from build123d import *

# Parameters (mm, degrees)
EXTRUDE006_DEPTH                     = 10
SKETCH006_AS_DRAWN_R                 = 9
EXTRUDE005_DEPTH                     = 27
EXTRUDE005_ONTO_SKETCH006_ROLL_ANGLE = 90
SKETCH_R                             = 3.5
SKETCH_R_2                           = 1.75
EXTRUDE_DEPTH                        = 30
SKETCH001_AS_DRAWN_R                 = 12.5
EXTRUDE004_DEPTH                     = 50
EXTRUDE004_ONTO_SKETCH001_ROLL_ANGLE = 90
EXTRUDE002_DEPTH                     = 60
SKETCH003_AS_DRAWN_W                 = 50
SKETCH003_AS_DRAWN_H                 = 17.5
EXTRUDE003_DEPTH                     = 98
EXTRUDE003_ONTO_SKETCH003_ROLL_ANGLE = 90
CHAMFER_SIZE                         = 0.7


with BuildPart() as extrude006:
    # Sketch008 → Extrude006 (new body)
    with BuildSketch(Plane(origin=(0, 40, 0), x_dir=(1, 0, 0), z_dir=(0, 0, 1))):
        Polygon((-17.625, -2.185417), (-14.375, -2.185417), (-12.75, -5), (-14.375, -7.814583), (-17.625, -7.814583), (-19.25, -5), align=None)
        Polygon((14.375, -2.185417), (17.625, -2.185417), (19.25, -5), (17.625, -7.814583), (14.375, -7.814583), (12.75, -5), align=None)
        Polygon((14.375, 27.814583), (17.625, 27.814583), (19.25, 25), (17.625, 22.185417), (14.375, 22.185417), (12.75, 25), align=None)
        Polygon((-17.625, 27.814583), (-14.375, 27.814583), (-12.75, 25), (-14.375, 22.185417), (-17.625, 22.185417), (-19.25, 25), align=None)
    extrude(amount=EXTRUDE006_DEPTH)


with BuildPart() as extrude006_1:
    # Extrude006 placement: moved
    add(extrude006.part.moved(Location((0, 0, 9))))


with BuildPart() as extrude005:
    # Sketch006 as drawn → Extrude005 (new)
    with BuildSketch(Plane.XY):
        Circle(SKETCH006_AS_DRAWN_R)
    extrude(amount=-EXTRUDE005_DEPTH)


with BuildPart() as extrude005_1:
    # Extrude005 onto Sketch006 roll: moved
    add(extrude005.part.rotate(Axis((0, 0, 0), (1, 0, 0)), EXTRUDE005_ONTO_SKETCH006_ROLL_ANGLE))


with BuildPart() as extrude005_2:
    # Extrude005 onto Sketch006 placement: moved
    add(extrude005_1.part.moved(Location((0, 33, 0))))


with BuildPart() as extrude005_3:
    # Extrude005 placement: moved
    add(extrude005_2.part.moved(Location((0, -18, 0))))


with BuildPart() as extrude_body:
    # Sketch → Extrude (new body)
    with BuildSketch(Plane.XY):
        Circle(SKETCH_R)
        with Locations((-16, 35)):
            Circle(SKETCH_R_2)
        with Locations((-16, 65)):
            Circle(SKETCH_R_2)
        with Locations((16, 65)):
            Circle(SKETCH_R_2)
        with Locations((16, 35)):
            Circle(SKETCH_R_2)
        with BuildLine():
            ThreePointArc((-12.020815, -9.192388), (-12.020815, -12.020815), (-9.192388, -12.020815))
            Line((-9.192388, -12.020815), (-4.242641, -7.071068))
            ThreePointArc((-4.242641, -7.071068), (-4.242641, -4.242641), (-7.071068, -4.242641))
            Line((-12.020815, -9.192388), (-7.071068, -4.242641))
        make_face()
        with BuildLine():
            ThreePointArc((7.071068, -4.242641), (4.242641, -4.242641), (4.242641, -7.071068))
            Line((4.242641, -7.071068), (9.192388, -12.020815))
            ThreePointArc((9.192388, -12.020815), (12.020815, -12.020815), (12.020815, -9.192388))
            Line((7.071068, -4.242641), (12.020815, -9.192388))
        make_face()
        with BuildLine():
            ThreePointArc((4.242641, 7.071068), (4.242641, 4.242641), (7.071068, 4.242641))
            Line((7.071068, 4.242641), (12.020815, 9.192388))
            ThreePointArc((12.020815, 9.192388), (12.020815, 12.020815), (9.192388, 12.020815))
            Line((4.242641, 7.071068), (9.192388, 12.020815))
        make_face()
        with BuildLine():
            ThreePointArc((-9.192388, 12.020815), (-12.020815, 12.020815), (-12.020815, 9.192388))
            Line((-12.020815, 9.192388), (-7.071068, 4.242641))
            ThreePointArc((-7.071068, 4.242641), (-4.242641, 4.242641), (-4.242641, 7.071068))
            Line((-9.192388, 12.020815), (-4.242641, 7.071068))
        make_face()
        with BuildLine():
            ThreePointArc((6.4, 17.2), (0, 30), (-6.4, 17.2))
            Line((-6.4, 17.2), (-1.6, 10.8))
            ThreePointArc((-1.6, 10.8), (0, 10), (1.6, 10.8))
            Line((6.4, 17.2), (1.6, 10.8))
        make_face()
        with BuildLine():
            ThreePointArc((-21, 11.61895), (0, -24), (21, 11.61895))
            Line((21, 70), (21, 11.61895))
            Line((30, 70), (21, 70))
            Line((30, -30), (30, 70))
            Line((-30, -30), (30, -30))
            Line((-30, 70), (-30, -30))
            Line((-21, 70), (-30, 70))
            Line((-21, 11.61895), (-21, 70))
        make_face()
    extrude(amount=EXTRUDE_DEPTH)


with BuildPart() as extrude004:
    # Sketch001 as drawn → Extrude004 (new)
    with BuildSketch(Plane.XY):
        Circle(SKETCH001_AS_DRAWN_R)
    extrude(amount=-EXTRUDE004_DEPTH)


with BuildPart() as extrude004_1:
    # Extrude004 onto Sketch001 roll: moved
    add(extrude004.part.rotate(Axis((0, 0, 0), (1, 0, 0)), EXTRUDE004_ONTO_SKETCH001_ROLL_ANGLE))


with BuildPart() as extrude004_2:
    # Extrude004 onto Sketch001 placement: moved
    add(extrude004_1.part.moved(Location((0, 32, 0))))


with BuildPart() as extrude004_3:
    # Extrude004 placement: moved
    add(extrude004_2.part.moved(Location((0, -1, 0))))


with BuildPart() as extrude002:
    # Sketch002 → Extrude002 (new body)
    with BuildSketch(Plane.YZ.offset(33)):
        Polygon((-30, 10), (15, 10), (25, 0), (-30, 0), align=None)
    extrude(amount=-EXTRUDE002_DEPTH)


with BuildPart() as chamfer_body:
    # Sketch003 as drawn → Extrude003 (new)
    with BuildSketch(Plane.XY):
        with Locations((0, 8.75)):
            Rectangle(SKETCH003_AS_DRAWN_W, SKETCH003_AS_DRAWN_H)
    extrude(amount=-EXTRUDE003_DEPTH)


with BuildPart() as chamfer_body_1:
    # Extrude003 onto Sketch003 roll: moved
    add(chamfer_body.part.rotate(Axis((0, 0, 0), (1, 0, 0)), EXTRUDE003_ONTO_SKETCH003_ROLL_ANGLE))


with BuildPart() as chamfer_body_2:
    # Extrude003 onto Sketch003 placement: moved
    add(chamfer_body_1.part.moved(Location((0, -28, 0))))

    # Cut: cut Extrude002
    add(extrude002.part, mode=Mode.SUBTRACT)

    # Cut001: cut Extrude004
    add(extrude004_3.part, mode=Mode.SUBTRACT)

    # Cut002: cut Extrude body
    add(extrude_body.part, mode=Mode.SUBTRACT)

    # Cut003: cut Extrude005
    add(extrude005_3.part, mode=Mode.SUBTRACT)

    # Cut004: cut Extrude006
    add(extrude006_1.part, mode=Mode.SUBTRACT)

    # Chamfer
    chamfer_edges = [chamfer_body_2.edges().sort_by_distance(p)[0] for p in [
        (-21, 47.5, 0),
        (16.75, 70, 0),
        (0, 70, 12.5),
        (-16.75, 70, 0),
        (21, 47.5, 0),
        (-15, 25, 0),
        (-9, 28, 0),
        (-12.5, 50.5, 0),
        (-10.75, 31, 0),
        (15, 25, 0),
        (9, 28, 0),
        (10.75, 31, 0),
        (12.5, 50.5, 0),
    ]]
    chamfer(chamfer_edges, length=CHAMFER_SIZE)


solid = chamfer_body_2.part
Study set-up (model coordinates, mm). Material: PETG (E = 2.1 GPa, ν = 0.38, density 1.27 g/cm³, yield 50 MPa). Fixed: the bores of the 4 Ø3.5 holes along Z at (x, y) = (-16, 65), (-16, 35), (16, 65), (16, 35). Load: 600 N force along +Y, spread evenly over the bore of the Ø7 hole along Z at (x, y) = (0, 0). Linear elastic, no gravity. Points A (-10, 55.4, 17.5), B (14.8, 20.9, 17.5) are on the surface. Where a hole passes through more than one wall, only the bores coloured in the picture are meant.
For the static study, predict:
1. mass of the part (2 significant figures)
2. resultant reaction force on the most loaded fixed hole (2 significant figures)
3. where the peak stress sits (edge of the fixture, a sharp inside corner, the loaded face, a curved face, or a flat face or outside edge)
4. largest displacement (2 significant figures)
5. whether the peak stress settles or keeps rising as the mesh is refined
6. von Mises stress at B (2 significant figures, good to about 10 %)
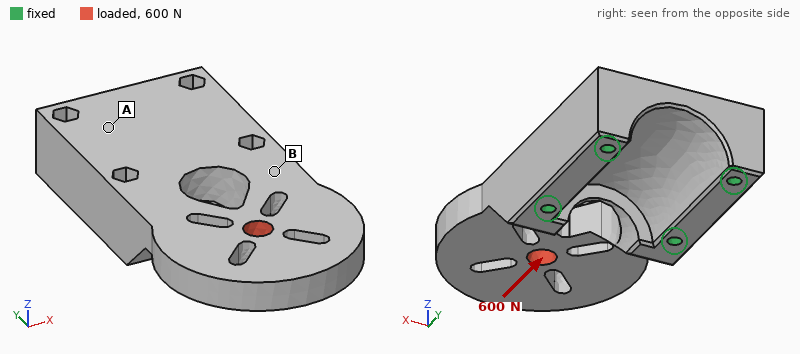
44 g
200 N
edge of the fixture
0.29 mm
keeps rising
3.0 MPa
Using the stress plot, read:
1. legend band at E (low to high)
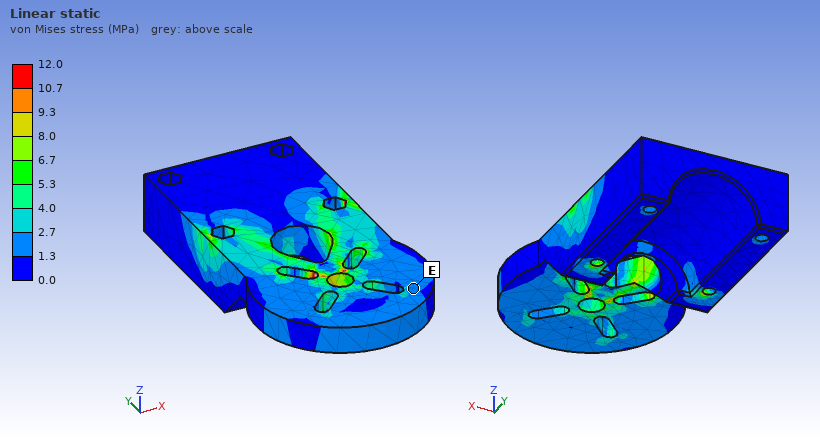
1.3 to 2.7 MPa
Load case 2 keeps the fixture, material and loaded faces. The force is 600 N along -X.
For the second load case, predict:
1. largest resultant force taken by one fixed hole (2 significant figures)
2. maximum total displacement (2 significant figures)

530 N
0.50 mm
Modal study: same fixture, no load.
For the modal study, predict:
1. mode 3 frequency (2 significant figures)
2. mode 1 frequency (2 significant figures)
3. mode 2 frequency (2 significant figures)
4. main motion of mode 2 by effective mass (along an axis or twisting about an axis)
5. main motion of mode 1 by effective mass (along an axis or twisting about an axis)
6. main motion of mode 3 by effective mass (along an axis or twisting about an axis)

1800 Hz
660 Hz
1400 Hz
along X
along Z
along X
